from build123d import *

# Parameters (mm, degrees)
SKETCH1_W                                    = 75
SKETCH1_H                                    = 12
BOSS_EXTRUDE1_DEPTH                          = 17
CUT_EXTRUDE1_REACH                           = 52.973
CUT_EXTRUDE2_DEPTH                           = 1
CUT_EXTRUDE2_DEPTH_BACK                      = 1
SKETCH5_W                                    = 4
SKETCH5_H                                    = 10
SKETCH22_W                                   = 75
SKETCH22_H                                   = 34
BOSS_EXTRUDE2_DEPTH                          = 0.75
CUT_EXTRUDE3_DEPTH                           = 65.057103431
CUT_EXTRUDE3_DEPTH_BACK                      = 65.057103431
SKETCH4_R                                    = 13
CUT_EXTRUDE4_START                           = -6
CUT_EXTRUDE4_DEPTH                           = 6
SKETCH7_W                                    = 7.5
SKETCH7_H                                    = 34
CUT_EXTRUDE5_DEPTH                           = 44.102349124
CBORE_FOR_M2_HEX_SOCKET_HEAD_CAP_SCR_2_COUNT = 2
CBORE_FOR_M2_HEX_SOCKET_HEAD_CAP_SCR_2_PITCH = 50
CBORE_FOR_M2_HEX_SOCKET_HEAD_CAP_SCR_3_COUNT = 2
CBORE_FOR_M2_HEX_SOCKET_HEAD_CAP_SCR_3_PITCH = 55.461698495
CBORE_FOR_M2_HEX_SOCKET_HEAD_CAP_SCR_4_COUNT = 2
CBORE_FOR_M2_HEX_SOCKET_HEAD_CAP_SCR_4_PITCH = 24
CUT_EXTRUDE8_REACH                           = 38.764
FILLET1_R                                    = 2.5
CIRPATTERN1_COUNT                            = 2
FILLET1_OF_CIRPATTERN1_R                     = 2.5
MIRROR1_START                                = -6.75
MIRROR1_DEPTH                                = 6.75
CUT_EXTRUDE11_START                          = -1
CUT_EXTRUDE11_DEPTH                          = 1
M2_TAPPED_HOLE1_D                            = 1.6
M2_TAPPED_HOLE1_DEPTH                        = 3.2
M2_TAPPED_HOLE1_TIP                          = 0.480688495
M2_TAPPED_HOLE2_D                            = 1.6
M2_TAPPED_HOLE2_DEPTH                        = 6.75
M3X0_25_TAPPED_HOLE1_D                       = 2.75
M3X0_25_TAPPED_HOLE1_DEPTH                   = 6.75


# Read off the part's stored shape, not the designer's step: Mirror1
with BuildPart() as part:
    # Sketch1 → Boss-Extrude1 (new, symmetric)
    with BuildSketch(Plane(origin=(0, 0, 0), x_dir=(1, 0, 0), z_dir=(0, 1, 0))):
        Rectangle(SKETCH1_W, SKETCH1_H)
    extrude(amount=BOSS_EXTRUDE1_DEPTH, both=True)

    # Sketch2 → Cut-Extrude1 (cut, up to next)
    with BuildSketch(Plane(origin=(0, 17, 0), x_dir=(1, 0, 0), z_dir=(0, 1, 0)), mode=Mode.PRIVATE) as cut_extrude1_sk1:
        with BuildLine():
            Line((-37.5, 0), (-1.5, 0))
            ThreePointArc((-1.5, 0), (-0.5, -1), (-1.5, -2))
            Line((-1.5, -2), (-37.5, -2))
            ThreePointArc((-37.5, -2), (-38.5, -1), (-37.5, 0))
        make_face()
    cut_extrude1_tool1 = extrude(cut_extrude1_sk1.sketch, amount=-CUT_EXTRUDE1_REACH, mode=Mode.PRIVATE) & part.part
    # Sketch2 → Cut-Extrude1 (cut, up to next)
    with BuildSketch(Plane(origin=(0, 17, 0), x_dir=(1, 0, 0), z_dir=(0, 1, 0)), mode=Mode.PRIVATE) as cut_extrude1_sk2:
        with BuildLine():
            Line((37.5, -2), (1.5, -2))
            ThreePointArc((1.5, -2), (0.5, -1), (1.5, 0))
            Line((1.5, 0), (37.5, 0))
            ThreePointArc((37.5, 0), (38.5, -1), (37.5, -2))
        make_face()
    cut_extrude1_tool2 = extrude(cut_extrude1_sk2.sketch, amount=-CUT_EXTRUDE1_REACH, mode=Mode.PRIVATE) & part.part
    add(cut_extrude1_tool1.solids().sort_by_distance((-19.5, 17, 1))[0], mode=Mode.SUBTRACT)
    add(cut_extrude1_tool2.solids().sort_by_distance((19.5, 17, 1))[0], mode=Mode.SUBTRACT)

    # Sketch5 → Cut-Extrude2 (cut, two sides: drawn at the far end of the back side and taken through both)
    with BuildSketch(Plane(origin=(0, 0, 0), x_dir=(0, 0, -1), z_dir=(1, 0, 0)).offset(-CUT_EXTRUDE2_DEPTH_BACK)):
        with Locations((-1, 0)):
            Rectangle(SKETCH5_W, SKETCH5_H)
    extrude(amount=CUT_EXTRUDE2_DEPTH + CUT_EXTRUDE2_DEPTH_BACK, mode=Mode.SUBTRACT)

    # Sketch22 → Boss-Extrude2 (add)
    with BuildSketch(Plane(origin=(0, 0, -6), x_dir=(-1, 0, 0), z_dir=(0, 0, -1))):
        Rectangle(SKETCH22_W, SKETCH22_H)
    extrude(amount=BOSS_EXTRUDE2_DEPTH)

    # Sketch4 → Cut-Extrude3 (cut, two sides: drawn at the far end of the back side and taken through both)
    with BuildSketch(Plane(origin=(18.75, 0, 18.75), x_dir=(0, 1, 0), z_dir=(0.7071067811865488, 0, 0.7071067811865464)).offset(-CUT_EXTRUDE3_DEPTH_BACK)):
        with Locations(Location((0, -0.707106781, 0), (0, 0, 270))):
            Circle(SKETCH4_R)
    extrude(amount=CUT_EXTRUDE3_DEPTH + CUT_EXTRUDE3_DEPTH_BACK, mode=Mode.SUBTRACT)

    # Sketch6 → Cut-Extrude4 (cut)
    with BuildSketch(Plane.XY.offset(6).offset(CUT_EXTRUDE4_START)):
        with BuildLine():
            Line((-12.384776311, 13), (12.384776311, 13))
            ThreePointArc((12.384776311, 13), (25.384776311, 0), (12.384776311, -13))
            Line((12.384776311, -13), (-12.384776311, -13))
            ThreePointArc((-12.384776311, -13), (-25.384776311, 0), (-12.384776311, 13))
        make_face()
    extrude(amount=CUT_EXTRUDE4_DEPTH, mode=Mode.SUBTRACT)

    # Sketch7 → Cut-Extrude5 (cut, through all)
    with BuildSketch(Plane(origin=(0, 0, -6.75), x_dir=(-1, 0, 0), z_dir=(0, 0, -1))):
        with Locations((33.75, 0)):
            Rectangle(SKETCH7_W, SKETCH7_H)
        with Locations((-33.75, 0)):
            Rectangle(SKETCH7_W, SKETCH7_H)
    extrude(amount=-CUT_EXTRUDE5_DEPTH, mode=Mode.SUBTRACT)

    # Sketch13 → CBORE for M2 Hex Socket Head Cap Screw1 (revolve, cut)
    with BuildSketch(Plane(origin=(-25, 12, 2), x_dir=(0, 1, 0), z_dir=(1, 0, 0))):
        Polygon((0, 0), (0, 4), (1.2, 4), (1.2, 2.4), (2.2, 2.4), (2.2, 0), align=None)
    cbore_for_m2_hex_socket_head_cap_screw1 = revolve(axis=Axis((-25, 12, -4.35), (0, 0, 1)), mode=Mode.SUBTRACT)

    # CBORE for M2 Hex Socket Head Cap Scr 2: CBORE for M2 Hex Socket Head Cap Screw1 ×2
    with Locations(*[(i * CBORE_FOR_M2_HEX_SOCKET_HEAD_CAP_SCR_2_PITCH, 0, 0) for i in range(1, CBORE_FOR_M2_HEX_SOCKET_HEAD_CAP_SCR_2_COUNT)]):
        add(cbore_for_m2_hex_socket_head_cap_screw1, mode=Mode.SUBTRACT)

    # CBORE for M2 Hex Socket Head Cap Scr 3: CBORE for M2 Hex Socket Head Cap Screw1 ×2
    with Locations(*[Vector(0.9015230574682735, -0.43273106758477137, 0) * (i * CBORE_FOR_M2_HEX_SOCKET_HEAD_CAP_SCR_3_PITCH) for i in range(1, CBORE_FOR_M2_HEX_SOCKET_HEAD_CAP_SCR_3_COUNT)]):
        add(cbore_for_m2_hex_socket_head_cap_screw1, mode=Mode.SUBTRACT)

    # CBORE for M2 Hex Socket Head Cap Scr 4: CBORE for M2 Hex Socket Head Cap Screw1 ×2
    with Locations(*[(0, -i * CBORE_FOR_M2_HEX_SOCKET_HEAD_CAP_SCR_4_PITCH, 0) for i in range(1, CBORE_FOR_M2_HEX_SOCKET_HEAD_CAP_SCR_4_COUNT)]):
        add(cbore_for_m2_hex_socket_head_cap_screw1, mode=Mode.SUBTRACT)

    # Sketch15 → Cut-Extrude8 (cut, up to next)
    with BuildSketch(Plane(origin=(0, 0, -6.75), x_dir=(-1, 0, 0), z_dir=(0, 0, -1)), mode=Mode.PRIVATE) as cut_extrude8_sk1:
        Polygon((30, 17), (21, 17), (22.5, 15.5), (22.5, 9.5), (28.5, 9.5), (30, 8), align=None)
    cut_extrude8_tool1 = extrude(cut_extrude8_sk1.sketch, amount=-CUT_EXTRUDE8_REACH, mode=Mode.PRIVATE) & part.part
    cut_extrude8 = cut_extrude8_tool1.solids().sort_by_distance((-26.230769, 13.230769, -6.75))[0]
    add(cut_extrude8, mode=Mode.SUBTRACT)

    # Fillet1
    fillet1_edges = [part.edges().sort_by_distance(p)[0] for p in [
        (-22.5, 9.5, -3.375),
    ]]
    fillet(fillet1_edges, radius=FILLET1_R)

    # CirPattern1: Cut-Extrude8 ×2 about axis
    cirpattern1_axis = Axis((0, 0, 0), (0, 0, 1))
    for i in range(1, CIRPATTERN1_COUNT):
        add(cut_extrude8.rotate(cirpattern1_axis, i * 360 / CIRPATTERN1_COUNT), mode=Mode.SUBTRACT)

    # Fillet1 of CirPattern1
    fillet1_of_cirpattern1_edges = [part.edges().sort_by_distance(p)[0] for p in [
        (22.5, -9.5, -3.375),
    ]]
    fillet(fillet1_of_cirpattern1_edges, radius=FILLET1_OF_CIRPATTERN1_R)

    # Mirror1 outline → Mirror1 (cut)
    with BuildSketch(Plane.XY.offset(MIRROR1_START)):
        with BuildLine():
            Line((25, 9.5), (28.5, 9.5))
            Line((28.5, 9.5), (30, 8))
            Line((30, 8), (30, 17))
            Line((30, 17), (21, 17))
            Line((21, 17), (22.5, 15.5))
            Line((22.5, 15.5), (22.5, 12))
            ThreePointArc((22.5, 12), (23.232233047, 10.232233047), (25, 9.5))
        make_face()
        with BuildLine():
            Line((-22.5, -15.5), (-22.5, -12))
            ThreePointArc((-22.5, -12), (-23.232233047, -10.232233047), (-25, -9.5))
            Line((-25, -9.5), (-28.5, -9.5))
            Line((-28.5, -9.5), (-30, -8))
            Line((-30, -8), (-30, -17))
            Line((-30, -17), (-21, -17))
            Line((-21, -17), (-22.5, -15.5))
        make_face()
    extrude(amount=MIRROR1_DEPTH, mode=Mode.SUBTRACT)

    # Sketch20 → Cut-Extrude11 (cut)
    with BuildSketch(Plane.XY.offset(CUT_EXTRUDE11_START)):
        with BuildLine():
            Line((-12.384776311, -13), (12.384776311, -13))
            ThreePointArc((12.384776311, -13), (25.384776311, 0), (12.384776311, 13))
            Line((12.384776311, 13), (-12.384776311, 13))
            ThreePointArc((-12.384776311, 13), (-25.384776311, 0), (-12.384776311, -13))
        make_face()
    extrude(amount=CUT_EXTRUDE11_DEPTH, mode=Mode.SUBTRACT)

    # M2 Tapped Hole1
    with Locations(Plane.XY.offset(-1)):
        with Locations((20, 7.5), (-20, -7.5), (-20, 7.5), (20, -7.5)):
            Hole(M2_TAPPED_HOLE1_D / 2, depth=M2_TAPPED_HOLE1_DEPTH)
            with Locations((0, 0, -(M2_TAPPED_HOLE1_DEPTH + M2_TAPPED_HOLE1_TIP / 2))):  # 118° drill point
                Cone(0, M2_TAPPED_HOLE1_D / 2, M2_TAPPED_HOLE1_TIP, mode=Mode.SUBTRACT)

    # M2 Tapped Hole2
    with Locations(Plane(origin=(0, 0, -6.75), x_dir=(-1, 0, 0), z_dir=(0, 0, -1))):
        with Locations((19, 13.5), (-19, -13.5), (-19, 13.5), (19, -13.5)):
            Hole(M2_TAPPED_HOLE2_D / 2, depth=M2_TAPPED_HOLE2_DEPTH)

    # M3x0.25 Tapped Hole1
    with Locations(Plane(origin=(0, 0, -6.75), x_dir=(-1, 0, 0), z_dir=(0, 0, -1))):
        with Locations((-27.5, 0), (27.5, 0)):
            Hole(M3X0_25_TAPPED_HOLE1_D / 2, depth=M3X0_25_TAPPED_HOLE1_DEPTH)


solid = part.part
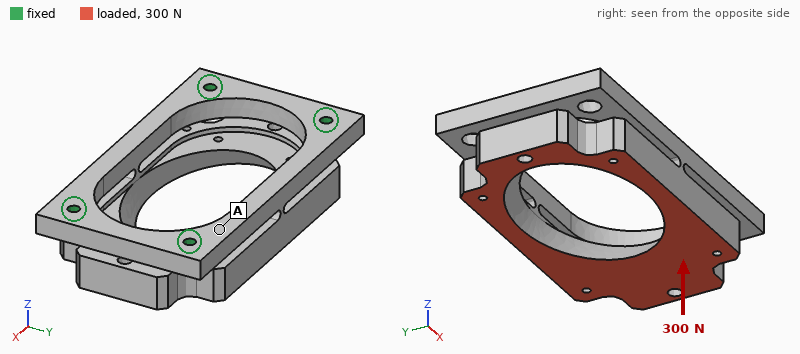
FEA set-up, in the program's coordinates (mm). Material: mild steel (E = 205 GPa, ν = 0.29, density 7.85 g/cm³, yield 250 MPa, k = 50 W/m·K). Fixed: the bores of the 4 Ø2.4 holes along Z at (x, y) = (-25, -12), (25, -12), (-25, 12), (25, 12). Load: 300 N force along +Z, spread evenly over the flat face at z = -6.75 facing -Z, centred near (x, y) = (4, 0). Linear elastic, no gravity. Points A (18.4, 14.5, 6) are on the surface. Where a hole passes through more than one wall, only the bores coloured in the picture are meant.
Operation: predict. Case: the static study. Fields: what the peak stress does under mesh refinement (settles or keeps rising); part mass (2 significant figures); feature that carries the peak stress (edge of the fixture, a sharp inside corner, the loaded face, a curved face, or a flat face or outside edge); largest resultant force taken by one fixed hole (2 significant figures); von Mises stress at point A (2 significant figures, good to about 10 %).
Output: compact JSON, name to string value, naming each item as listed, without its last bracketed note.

{"what the peak stress does under mesh refinement": "keeps rising", "part mass": "78 g", "feature that carries the peak stress": "a sharp inside corner", "largest resultant force taken by one fixed hole": "140 N", "von Mises stress at point A": "34 MPa"}
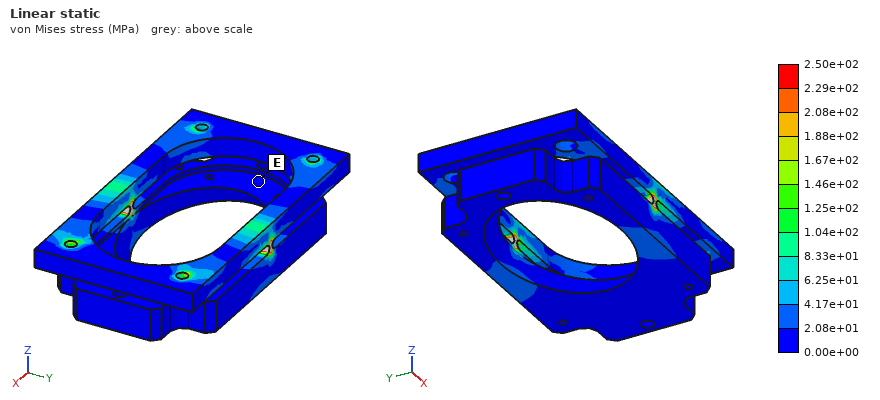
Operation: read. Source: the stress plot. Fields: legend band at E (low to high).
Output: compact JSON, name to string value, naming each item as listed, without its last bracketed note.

{"legend band at E": "0.00e+00 to 2.08e+01 MPa"}
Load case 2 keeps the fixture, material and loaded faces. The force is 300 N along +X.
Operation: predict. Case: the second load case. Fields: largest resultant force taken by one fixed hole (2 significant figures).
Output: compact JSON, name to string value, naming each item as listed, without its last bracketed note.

{"largest resultant force taken by one fixed hole": "90 N"}
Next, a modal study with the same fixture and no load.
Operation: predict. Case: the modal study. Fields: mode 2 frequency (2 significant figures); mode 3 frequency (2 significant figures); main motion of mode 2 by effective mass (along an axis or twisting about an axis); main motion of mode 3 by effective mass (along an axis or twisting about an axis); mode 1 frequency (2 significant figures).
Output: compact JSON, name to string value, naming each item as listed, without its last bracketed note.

{"mode 2 frequency": "2000 Hz", "mode 3 frequency": "2200 Hz", "main motion of mode 2 by effective mass": "along Z", "main motion of mode 3 by effective mass": "along Y", "mode 1 frequency": "350 Hz"}
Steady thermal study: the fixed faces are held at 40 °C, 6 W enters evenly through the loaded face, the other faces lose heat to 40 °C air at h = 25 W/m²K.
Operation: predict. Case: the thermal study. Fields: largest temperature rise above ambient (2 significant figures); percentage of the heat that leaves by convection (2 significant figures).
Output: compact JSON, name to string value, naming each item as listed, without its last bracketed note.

{"largest temperature rise above ambient": "44 K", "percentage of the heat that leaves by convection": "61 %"}
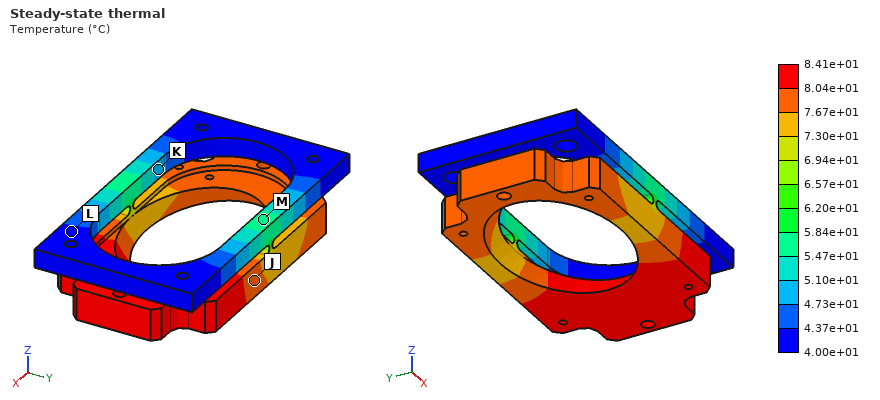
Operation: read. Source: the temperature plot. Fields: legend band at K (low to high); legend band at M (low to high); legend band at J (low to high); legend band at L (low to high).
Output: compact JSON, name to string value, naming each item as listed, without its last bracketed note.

{"legend band at K": "4.73e+01 to 5.10e+01 °C", "legend band at M": "5.47e+01 to 5.84e+01 °C", "legend band at J": "7.67e+01 to 8.04e+01 °C", "legend band at L": "4.00e+01 to 4.37e+01 °C"}
